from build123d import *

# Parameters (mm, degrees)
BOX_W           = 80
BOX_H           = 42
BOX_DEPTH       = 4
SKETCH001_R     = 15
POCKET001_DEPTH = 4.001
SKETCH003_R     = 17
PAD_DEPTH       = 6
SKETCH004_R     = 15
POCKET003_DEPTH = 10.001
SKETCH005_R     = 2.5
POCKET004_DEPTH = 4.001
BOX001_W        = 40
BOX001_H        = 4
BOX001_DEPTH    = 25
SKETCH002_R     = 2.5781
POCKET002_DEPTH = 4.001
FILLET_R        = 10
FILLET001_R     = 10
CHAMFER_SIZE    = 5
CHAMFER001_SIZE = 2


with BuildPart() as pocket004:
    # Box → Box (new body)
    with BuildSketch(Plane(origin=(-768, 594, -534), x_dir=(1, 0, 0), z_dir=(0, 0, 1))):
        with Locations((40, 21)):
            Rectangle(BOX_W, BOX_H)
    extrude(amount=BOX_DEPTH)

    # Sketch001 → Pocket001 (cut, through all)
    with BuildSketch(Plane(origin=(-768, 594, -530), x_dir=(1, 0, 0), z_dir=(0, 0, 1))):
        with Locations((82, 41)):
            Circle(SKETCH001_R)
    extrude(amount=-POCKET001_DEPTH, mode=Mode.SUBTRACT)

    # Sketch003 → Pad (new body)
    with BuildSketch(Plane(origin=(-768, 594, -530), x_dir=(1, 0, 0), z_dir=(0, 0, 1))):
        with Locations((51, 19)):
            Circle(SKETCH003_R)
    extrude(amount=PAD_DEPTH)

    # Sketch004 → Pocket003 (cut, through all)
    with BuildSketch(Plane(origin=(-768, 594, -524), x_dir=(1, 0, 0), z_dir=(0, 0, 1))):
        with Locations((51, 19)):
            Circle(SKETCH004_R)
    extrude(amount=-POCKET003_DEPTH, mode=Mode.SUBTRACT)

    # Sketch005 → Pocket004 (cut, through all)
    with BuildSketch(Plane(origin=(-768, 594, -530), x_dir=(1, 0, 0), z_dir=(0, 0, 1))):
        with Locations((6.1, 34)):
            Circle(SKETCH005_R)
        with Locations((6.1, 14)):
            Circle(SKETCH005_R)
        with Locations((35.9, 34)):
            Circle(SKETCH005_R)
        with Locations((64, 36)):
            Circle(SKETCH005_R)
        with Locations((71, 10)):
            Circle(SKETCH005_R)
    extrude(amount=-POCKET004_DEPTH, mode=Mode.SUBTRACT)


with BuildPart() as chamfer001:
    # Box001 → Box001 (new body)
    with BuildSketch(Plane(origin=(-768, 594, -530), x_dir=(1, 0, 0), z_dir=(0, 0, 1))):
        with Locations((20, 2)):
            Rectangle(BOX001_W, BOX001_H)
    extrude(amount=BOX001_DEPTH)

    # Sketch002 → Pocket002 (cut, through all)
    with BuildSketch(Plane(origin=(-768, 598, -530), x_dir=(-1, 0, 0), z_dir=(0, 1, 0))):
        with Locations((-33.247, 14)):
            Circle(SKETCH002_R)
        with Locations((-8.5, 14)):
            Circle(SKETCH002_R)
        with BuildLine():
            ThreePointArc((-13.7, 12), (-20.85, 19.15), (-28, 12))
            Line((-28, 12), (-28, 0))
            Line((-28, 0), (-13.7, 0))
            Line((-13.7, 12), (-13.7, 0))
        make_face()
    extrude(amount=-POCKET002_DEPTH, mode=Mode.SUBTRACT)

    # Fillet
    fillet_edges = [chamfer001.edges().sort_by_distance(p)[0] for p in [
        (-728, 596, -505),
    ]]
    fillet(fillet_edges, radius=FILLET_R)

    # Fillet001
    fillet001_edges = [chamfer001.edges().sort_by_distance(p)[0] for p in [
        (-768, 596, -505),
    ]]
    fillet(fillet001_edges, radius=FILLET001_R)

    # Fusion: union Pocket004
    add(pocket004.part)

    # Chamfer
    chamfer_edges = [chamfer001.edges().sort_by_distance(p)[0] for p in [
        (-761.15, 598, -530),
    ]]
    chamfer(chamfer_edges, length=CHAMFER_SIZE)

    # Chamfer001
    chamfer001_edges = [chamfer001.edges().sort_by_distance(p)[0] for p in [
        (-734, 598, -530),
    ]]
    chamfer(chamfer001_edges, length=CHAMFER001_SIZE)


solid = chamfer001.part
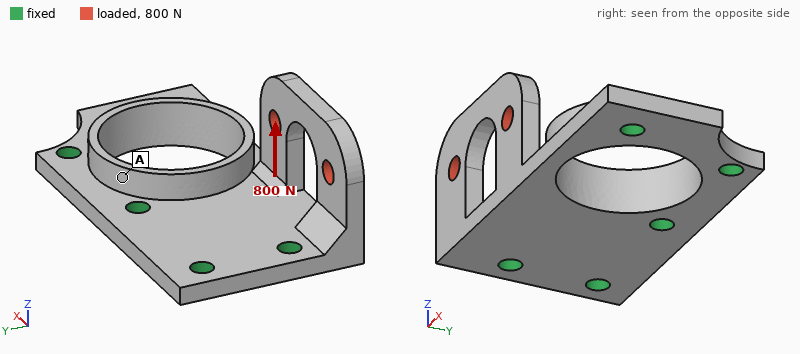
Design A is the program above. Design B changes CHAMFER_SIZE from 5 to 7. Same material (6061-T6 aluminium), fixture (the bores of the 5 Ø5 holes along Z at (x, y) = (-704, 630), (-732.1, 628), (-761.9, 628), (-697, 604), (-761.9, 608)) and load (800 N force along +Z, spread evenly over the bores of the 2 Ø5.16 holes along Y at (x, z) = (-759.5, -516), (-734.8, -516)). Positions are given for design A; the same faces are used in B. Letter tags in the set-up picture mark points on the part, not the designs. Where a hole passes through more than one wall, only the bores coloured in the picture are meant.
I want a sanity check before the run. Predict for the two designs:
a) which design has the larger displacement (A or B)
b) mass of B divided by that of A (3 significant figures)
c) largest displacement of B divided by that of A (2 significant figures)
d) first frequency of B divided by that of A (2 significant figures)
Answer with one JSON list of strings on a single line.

["A", "1.01", "0.91", "1.1"]
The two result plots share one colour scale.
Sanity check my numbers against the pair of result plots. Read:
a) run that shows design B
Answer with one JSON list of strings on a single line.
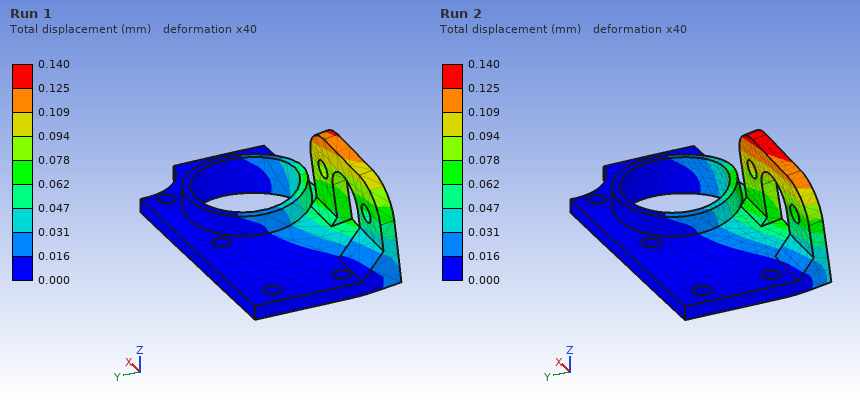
["Run 1"]
